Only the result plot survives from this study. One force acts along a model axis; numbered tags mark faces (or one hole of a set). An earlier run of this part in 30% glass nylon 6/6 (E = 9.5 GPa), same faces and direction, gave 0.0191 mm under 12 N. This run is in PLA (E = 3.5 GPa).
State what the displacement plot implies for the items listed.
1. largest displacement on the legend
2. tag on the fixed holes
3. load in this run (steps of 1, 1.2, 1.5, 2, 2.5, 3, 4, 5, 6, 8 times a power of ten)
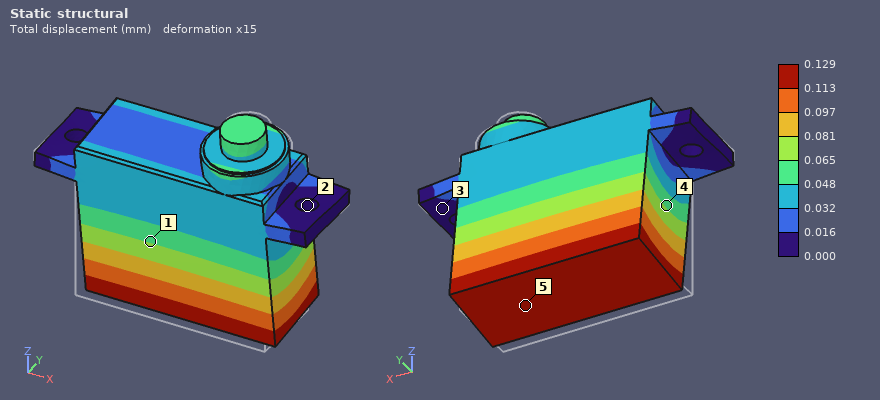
0.129 mm
2
30 N
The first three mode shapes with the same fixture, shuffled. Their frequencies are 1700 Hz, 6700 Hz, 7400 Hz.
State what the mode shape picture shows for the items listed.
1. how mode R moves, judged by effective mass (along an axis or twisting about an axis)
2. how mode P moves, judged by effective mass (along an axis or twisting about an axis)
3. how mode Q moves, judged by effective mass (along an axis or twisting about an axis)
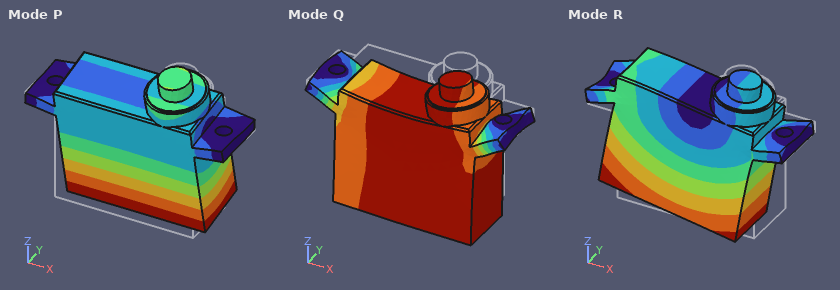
along X
along Y
along Z
